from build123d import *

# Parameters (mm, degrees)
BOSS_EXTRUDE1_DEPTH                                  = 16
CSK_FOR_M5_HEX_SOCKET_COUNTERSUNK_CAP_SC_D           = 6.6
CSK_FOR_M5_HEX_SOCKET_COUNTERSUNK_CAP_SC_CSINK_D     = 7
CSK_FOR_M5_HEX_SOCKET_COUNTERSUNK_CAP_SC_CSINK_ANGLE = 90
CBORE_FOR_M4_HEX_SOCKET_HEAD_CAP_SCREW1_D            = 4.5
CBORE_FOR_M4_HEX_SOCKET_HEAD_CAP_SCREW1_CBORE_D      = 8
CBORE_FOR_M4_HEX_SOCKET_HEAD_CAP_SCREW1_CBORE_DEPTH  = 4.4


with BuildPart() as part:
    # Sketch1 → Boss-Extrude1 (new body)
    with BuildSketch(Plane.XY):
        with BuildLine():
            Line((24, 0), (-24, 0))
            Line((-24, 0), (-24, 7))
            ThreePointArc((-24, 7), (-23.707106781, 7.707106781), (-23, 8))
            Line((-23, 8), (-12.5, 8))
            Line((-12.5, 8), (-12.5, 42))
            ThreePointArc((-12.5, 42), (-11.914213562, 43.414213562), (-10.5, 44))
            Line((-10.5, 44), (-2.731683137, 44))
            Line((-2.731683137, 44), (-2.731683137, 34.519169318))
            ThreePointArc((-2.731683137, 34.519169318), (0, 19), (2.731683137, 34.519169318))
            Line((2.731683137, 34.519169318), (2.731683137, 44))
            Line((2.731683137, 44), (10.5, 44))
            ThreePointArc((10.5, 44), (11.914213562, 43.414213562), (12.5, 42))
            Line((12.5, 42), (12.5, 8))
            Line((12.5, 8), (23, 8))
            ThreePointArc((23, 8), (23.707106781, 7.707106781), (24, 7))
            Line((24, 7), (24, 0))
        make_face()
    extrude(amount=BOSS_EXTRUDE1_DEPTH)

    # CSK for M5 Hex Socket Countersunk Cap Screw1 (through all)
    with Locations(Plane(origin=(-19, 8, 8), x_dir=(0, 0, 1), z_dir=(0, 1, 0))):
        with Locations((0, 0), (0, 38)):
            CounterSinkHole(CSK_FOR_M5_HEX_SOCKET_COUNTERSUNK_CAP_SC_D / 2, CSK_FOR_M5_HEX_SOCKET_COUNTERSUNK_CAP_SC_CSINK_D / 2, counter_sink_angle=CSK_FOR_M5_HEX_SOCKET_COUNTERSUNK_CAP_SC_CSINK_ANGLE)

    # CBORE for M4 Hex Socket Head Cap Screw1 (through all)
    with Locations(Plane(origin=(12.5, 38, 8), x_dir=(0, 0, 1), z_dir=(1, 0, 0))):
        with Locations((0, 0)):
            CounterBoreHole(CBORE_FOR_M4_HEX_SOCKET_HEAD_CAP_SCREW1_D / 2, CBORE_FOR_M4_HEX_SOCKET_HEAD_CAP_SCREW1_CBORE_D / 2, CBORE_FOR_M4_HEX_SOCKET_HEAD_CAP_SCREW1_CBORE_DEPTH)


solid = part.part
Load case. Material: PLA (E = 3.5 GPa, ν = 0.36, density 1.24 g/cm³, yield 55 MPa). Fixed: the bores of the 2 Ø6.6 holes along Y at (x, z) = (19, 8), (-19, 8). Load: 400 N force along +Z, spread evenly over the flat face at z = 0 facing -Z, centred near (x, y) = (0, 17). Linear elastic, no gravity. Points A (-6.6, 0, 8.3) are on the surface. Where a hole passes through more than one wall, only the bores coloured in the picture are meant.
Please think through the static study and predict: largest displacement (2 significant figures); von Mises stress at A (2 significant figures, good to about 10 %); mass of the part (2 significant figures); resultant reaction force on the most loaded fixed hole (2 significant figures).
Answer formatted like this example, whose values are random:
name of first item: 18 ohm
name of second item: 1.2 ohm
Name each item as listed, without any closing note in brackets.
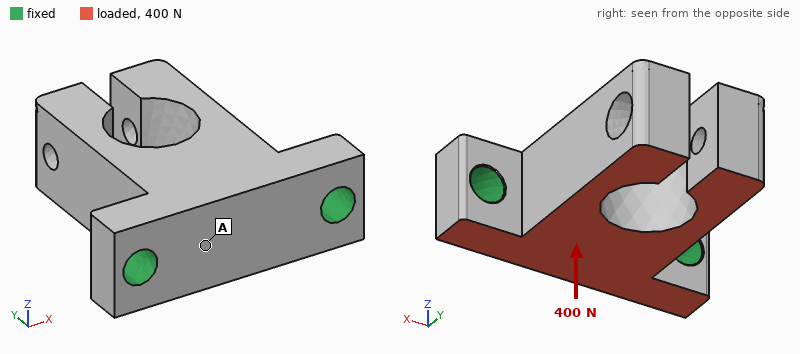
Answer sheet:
largest displacement: 0.39 mm
von Mises stress at A: 2.7 MPa
mass of the part: 19 g
resultant reaction force on the most loaded fixed hole: 200 N
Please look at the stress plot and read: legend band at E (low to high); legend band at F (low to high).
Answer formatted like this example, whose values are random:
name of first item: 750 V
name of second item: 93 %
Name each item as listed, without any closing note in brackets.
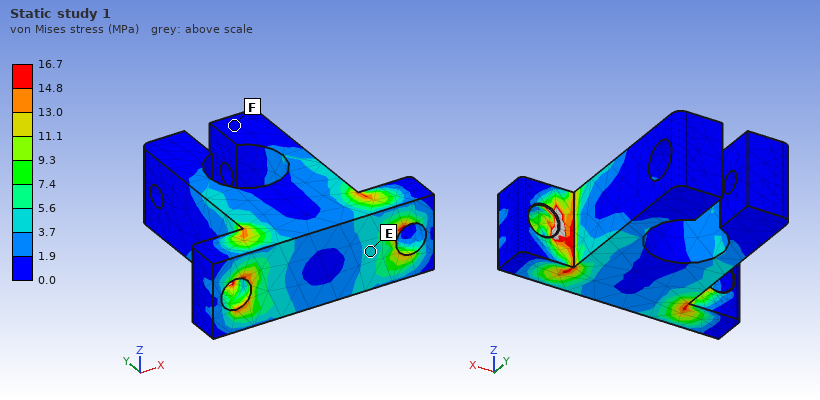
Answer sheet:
legend band at E: 3.7 to 5.6 MPa
legend band at F: 0.0 to 1.9 MPa
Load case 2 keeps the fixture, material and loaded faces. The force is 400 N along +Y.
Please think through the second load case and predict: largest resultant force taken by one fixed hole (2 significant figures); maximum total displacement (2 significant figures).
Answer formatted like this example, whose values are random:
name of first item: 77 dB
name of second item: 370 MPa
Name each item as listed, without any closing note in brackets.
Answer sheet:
largest resultant force taken by one fixed hole: 210 N
maximum total displacement: 0.21 mm
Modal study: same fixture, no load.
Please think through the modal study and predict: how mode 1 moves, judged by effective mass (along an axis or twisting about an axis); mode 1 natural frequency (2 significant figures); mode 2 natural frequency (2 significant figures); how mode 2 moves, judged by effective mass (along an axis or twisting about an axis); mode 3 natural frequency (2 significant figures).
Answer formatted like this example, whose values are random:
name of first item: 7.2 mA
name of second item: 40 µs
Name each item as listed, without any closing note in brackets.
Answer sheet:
how mode 1 moves, judged by effective mass: along Z
mode 1 natural frequency: 1500 Hz
mode 2 natural frequency: 1600 Hz
how mode 2 moves, judged by effective mass: along X
mode 3 natural frequency: 1700 Hz
